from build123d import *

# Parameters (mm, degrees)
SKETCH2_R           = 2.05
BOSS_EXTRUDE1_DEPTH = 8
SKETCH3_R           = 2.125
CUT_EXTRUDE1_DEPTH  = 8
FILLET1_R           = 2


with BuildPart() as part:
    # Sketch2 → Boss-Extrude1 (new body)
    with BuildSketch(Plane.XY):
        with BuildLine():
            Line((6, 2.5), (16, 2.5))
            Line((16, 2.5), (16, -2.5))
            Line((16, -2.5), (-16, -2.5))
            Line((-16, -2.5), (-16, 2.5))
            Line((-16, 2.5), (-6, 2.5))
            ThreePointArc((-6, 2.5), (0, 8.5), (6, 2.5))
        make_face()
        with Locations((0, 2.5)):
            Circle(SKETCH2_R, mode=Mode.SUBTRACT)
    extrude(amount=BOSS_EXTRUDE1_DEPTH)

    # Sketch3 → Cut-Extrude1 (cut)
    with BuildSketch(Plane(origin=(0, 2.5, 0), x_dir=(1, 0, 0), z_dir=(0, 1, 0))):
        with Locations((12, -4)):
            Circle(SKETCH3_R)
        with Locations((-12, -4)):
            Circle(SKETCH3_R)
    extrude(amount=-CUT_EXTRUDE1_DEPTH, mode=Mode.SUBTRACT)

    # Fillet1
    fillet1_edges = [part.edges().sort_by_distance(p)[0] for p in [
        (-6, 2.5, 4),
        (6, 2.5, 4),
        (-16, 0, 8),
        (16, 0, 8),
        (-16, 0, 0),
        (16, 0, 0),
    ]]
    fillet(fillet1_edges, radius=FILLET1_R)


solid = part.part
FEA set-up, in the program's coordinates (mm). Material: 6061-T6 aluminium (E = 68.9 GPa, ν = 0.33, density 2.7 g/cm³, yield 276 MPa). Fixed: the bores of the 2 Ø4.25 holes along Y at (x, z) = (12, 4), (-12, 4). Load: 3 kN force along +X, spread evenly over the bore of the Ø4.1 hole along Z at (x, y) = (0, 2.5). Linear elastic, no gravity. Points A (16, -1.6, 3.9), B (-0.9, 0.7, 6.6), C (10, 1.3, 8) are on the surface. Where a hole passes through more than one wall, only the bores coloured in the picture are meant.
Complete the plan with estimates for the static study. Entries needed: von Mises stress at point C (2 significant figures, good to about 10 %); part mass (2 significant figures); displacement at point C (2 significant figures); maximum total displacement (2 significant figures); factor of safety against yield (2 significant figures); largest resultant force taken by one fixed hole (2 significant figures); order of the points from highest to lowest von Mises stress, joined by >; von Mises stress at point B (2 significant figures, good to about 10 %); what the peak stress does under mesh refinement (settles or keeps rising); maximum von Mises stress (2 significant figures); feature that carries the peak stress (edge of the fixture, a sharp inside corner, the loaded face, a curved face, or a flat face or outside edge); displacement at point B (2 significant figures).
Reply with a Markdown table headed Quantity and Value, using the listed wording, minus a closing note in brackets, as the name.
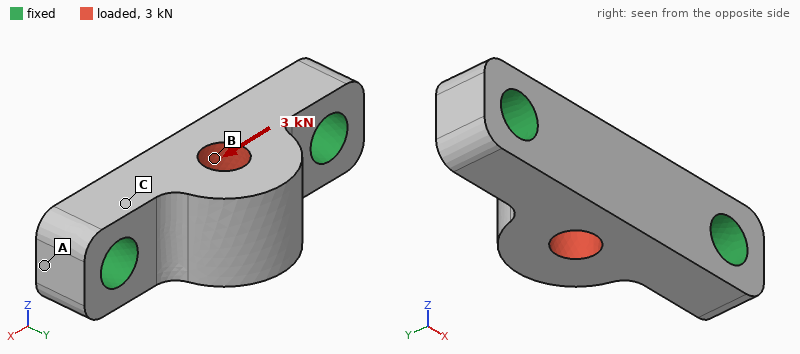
| Quantity | Value |
|---|---|
| von Mises stress at point C | 27 MPa |
| part mass | 4.0 g |
| displacement at point C | 1.5 µm |
| maximum total displacement | 8.4 µm |
| factor of safety against yield | 2.5 |
| largest resultant force taken by one fixed hole | 1.5 kN |
| order of the points from highest to lowest von Mises stress, joined by > | B > C > A |
| von Mises stress at point B | 49 MPa |
| what the peak stress does under mesh refinement | settles |
| maximum von Mises stress | 110 MPa |
| feature that carries the peak stress | a curved face |
| displacement at point B | 4.6 µm |
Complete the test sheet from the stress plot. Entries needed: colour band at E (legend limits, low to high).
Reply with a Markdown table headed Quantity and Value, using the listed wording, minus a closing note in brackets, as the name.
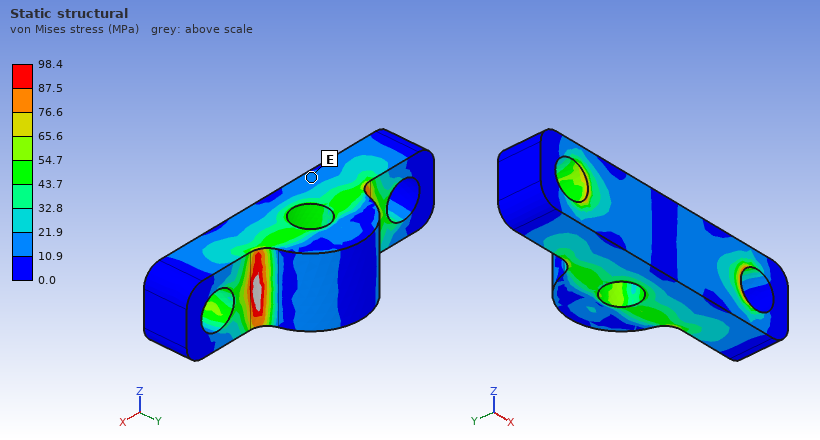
| Quantity | Value |
|---|---|
| colour band at E | 10.9 to 21.9 MPa |
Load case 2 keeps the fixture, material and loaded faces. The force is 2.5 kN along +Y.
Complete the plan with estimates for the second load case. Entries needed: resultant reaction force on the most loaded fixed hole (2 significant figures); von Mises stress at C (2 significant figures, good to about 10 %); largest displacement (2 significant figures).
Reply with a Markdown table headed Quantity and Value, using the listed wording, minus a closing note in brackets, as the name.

| Quantity | Value |
|---|---|
| resultant reaction force on the most loaded fixed hole | 1.3 kN |
| von Mises stress at C | 23 MPa |
| largest displacement | 20 µm |
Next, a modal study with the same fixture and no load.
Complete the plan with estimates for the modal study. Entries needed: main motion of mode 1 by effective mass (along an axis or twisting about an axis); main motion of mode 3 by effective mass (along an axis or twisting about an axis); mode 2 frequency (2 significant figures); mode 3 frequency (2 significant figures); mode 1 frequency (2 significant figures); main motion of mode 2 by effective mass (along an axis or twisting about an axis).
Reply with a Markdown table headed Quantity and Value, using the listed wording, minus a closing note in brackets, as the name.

| Quantity | Value |
|---|---|
| main motion of mode 1 by effective mass | along Z |
| main motion of mode 3 by effective mass | along Z |
| mode 2 frequency | 43 kHz |
| mode 3 frequency | 52 kHz |
| mode 1 frequency | 28 kHz |
| main motion of mode 2 by effective mass | along Y |
